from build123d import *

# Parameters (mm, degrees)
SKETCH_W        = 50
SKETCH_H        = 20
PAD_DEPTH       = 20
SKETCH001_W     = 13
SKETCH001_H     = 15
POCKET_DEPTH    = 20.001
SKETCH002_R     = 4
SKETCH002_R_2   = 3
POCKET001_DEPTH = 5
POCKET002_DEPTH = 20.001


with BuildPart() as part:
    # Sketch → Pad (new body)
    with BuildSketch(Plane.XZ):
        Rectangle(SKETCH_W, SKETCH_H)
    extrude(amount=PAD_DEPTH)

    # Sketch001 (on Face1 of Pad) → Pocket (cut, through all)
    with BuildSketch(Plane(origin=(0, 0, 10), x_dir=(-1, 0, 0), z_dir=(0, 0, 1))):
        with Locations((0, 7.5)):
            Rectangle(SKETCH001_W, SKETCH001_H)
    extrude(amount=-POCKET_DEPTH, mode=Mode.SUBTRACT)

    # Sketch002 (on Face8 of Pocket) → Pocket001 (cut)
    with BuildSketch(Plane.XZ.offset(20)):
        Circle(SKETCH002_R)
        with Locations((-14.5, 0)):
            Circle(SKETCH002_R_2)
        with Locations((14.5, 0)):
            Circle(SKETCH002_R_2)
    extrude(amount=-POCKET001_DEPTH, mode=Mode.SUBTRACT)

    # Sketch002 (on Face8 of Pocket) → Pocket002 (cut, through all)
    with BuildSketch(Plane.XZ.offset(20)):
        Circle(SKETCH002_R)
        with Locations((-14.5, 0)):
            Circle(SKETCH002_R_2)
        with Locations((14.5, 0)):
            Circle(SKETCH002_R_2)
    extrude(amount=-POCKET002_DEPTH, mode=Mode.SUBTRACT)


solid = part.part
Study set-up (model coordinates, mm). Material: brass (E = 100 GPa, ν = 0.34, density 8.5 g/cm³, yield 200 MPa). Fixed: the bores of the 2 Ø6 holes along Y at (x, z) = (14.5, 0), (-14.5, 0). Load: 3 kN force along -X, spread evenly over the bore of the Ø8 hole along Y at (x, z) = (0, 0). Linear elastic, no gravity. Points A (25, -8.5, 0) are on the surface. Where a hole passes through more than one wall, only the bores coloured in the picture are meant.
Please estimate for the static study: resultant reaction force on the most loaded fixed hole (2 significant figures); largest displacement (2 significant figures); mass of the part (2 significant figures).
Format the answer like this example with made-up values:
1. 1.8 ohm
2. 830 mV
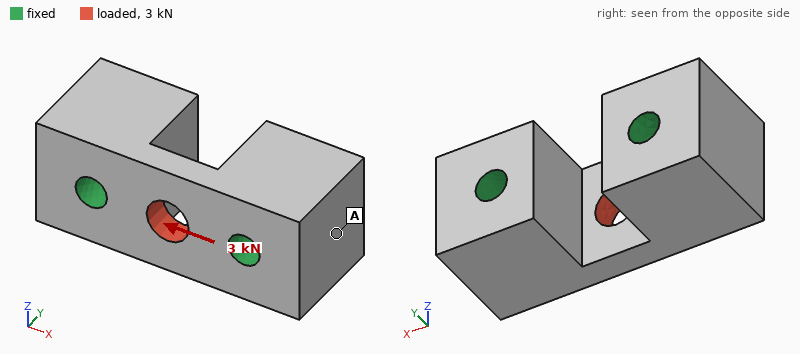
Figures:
1. 1.5 kN
2. 2.5 µm
3. 130 g
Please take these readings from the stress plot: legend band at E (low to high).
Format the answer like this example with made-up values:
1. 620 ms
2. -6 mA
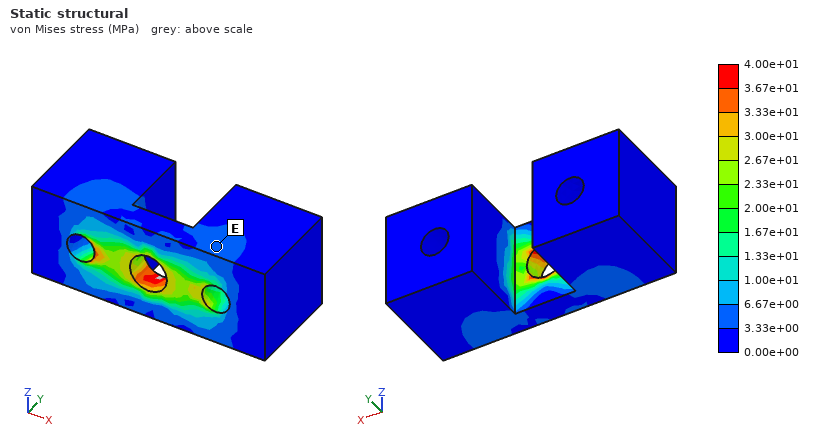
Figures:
1. 3.33e+00 to 6.67e+00 MPa
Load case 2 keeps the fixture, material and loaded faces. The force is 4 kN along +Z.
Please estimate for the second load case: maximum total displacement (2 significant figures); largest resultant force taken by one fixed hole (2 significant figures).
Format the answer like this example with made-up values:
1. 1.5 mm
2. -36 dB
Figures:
1. 8.3 µm
2. 2.0 kN
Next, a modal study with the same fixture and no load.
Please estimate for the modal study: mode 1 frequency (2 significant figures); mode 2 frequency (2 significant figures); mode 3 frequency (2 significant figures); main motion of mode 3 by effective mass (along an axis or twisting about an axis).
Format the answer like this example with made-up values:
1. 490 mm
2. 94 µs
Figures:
1. 27 kHz
2. 27 kHz
3. 37 kHz
4. along Y
